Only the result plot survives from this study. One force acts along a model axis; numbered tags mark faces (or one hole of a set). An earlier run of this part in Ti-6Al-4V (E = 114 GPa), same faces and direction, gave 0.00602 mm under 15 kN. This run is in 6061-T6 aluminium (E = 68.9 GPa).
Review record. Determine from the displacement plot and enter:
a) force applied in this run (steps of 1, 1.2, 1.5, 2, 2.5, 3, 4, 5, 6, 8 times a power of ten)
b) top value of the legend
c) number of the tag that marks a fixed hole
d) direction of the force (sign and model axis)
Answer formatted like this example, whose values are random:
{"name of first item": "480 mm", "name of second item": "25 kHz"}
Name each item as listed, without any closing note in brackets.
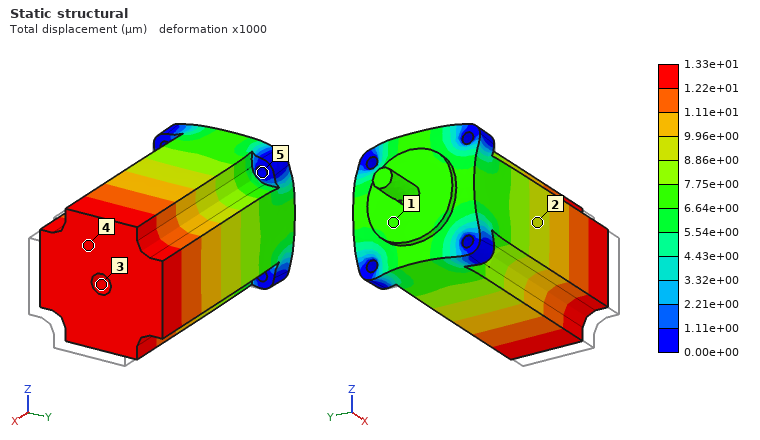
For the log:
{"force applied in this run": "20 kN", "top value of the legend": "1.33e+01 µm", "number of the tag that marks a fixed hole": "5", "direction of the force": "-X"}
